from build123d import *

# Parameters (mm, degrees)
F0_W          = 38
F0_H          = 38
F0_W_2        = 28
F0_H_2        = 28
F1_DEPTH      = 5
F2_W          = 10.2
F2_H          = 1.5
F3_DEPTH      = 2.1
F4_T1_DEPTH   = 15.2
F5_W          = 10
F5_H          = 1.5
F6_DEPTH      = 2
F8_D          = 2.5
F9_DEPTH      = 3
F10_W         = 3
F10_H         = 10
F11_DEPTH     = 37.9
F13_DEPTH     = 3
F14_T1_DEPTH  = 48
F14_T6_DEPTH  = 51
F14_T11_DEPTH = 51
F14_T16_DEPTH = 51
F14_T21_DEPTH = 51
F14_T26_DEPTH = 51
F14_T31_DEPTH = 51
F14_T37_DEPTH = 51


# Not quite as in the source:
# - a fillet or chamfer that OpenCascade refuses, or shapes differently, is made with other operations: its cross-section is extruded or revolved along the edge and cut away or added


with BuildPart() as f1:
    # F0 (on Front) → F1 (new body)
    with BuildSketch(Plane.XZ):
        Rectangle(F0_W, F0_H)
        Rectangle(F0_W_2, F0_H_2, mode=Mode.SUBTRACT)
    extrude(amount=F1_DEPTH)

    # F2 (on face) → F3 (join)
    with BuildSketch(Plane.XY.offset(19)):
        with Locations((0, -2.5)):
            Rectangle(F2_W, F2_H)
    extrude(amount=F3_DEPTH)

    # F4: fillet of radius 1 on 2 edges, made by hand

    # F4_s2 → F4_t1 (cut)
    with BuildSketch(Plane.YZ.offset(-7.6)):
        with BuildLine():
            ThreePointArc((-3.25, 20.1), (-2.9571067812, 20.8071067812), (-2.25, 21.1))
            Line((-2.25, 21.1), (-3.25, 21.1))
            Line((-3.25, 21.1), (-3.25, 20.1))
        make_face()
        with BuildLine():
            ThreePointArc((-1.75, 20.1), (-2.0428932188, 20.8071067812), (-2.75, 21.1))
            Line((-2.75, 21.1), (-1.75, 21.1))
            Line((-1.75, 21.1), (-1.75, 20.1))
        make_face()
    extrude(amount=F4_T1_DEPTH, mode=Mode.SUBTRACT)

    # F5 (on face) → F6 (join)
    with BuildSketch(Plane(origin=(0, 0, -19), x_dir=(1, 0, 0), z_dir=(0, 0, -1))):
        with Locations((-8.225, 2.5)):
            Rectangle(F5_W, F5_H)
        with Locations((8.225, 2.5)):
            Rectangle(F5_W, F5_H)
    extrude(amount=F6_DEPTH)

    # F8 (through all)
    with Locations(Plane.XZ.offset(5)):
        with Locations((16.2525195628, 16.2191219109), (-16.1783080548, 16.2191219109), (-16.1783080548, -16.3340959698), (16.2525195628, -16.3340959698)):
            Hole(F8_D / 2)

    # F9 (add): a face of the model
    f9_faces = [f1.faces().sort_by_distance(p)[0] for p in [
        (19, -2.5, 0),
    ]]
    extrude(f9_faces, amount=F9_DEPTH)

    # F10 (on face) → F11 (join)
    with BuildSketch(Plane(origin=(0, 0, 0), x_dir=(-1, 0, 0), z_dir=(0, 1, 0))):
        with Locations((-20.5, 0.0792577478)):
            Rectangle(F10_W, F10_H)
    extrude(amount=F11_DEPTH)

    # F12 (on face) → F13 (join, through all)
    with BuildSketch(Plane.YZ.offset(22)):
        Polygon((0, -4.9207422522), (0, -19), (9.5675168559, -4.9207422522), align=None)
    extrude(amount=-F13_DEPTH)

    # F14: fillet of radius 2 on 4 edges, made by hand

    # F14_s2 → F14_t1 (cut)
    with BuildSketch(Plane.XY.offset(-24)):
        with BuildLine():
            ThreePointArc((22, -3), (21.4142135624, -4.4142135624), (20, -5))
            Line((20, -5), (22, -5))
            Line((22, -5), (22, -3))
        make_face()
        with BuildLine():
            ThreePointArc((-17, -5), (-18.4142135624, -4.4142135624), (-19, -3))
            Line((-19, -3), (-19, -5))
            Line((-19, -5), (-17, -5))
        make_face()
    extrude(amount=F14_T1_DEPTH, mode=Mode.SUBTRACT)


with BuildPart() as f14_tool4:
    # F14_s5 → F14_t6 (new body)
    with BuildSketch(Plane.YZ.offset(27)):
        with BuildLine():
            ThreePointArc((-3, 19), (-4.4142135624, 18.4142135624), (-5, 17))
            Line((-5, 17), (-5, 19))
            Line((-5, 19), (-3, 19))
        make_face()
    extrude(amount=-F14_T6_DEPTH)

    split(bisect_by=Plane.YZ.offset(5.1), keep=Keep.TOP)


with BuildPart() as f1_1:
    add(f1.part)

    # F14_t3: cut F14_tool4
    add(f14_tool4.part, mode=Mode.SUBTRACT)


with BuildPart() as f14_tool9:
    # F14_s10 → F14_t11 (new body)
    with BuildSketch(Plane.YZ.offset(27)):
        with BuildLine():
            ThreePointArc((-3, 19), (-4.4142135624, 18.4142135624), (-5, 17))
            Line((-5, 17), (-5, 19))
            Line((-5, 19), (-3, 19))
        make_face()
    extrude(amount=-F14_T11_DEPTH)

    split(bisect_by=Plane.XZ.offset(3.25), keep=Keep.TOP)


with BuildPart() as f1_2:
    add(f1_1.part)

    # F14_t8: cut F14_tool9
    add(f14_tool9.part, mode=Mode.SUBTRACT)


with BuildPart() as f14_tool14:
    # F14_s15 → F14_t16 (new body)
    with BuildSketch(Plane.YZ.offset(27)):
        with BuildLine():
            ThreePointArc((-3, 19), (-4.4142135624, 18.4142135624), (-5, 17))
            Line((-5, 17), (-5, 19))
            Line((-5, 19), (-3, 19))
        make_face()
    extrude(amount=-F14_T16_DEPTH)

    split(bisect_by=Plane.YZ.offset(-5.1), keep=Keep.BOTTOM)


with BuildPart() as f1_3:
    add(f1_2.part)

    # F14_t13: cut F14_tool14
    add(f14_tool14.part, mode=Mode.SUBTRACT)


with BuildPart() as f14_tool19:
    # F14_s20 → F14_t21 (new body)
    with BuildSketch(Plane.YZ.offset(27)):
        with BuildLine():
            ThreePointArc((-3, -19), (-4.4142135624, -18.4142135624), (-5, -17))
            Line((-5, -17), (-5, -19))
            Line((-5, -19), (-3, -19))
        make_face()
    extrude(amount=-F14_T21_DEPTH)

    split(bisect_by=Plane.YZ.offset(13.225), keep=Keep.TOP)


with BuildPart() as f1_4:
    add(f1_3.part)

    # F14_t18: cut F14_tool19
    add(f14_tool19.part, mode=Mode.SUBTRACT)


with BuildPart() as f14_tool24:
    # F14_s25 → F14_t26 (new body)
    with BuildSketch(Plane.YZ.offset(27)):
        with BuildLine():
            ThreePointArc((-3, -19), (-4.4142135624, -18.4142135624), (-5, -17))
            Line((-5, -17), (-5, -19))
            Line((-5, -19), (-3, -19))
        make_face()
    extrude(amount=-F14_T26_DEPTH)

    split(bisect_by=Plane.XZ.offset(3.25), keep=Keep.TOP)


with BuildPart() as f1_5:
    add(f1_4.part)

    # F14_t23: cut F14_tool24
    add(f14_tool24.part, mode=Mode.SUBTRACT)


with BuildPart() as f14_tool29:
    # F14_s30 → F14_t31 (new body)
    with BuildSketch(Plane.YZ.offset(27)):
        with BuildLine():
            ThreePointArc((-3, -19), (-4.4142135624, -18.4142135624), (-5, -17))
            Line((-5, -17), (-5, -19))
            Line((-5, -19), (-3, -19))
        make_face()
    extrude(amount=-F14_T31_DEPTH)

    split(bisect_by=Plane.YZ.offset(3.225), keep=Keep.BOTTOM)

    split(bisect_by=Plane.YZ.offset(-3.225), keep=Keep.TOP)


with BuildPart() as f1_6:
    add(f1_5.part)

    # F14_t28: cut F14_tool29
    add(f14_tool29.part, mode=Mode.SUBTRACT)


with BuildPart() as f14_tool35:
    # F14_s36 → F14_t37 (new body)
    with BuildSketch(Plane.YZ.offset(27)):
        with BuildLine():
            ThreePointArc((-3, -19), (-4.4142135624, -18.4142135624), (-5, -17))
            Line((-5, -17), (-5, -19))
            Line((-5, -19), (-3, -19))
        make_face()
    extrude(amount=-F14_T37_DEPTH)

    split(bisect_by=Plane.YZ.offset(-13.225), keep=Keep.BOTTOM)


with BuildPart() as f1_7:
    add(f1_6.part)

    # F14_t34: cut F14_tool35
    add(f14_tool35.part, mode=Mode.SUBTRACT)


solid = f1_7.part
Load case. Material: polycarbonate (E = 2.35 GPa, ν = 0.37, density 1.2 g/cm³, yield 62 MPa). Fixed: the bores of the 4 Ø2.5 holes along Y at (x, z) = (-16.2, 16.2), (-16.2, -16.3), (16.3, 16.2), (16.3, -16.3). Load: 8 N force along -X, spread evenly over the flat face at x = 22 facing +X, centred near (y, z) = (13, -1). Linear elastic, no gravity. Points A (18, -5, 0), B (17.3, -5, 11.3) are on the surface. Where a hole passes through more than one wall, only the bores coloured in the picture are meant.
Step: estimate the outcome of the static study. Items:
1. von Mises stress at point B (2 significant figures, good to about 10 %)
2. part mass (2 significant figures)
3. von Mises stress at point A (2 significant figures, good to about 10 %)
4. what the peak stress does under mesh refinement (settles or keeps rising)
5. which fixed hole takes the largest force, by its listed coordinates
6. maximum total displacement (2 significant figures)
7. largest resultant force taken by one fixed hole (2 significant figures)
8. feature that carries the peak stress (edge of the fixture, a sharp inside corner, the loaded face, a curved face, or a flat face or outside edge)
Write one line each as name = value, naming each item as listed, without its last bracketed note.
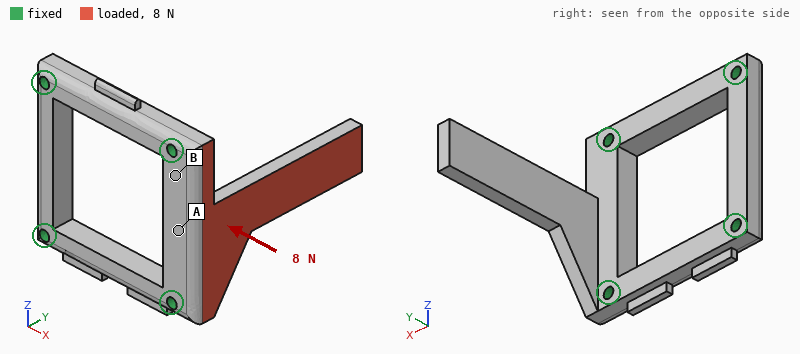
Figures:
von Mises stress at point B = 1.4 MPa
part mass = 6.1 g
von Mises stress at point A = 0.52 MPa
what the peak stress does under mesh refinement = keeps rising
which fixed hole takes the largest force, by its listed coordinates = (16.3, -16.3)
maximum total displacement = 0.77 mm
largest resultant force taken by one fixed hole = 5.2 N
feature that carries the peak stress = edge of the fixture
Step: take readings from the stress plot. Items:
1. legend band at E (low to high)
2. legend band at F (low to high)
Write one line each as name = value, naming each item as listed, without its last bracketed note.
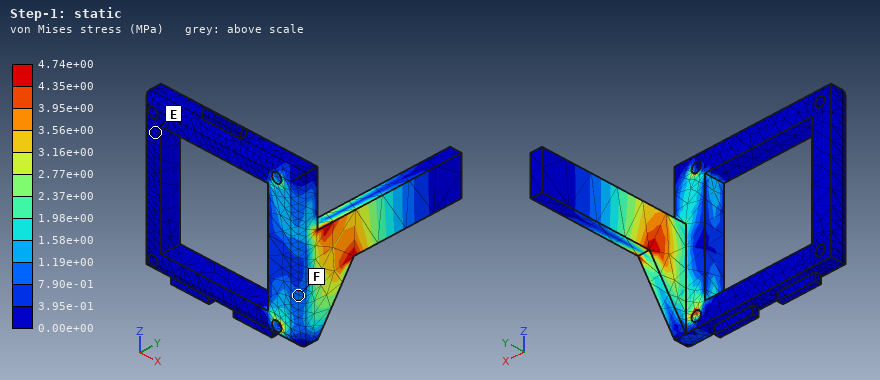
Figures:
legend band at E = 0.00e+00 to 3.95e-01 MPa
legend band at F = 7.90e-01 to 1.19e+00 MPa
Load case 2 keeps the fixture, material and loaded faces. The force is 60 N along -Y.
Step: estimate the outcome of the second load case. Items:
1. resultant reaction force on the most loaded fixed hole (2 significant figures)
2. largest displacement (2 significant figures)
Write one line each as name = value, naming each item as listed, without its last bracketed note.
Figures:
resultant reaction force on the most loaded fixed hole = 32 N
largest displacement = 0.79 mm
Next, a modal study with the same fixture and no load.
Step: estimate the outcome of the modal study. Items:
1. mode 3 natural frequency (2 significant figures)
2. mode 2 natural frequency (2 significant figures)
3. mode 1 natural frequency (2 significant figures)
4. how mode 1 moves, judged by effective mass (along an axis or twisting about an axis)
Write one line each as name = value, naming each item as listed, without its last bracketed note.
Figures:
mode 3 natural frequency = 2400 Hz
mode 2 natural frequency = 1600 Hz
mode 1 natural frequency = 460 Hz
how mode 1 moves, judged by effective mass = along X
